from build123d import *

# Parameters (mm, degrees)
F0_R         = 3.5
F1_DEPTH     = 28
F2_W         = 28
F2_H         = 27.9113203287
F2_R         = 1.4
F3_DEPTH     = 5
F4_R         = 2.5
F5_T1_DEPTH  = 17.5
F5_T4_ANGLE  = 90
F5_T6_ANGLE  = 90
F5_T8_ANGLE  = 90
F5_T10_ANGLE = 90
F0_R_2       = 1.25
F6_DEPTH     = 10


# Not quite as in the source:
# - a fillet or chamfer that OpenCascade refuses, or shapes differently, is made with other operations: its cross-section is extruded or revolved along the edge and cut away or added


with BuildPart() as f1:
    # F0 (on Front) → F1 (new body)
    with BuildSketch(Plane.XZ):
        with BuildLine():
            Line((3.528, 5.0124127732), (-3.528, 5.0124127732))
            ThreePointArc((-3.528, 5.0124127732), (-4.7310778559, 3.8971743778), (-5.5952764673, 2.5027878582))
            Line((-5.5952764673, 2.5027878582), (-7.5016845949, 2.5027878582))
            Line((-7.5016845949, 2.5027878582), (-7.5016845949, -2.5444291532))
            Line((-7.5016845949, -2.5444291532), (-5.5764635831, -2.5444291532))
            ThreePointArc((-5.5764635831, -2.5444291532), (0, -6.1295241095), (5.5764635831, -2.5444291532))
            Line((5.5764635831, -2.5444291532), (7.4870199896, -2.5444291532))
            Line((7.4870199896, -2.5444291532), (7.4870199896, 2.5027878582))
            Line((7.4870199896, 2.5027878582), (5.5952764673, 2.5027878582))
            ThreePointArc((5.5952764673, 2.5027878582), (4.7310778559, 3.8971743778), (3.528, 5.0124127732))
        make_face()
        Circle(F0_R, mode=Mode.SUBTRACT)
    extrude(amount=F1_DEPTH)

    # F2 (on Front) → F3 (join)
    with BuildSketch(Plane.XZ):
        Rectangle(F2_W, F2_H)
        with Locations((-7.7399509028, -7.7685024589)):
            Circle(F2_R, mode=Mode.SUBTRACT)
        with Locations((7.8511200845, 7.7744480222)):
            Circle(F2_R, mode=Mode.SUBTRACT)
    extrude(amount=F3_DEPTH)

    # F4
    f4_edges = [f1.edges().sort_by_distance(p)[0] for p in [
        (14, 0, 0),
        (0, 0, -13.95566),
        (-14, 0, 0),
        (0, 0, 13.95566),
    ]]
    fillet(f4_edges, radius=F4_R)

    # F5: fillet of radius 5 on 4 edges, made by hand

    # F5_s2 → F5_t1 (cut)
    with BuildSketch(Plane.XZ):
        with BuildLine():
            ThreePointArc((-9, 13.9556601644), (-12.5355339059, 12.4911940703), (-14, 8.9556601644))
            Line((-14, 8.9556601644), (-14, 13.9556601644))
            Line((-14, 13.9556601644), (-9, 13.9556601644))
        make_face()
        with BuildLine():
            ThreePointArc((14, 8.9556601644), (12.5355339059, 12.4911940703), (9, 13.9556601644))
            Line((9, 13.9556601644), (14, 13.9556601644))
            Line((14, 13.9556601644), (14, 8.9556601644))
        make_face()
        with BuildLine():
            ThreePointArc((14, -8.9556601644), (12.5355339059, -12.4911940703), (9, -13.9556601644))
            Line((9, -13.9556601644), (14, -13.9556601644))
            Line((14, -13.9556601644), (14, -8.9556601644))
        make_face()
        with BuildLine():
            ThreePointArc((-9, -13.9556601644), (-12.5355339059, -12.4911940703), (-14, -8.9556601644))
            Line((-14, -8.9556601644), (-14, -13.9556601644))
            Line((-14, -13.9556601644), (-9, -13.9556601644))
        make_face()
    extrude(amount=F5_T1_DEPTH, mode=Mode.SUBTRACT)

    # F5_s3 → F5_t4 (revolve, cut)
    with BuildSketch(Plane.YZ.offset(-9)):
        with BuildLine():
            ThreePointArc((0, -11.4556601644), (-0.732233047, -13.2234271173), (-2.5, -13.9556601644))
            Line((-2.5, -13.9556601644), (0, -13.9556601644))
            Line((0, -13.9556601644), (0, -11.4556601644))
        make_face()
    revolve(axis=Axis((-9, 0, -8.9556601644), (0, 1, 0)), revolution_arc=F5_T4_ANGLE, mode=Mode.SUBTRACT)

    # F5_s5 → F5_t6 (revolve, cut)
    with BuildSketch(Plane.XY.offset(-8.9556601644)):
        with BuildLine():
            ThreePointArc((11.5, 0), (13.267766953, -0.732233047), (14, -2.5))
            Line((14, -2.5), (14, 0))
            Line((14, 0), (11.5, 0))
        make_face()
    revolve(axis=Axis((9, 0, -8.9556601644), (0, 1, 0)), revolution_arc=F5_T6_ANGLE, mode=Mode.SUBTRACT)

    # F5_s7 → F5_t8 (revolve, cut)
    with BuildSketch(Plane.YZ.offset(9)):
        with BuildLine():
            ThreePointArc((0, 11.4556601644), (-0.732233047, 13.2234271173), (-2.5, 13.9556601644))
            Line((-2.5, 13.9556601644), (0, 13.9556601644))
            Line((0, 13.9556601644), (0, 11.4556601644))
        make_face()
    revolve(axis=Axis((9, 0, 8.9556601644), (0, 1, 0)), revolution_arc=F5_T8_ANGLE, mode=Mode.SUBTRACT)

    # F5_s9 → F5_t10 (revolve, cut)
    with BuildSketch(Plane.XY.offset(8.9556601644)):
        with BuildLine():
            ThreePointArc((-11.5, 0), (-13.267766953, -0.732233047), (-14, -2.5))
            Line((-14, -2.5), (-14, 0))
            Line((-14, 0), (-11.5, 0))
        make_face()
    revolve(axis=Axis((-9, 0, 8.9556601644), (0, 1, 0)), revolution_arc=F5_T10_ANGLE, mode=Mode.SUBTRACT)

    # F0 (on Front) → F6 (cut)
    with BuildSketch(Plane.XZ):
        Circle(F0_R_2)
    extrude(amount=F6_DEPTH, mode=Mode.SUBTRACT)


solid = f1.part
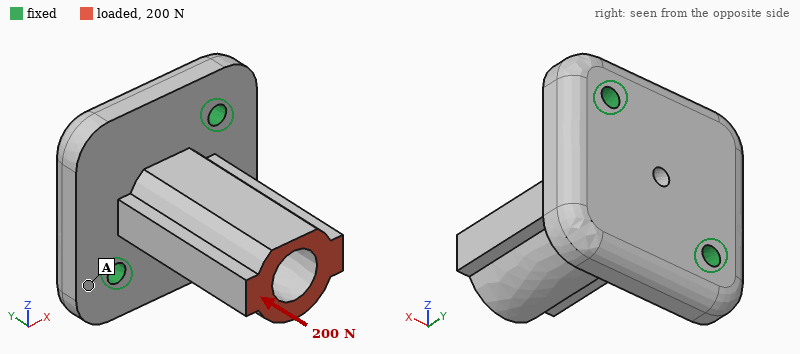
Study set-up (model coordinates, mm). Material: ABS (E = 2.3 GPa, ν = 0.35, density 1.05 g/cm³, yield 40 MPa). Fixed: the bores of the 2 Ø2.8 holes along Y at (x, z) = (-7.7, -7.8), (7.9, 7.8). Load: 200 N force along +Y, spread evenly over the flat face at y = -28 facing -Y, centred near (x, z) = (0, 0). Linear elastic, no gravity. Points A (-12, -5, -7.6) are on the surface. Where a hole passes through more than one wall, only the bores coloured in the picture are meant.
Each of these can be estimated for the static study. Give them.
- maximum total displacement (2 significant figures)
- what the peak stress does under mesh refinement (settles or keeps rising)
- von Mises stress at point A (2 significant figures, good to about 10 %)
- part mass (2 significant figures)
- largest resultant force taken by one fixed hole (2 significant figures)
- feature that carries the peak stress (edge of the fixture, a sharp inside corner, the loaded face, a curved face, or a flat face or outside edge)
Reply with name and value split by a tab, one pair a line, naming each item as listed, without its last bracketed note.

maximum total displacement	50 µm
what the peak stress does under mesh refinement	keeps rising
von Mises stress at point A	1.5 MPa
part mass	5.9 g
largest resultant force taken by one fixed hole	100 N
feature that carries the peak stress	edge of the fixture
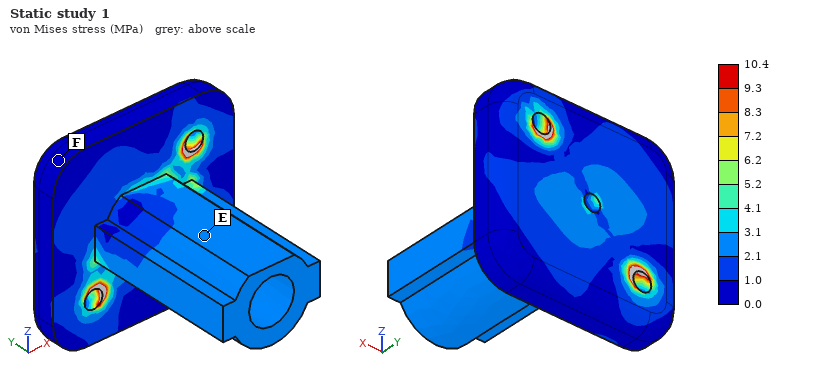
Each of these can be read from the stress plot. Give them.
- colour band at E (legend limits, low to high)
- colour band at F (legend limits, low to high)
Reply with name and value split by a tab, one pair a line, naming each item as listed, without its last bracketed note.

colour band at E	2.1 to 3.1 MPa
colour band at F	0.0 to 1.0 MPa
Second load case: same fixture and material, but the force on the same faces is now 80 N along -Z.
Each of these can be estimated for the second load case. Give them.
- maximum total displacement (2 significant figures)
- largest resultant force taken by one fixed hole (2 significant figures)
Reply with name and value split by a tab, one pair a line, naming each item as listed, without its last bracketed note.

maximum total displacement	0.49 mm
largest resultant force taken by one fixed hole	89 N
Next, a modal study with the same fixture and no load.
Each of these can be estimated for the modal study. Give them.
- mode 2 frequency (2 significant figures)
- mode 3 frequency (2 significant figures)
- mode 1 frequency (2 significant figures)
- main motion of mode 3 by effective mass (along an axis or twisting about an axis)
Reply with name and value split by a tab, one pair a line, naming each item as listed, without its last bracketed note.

mode 2 frequency	3400 Hz
mode 3 frequency	5300 Hz
mode 1 frequency	2000 Hz
main motion of mode 3 by effective mass	along Y
